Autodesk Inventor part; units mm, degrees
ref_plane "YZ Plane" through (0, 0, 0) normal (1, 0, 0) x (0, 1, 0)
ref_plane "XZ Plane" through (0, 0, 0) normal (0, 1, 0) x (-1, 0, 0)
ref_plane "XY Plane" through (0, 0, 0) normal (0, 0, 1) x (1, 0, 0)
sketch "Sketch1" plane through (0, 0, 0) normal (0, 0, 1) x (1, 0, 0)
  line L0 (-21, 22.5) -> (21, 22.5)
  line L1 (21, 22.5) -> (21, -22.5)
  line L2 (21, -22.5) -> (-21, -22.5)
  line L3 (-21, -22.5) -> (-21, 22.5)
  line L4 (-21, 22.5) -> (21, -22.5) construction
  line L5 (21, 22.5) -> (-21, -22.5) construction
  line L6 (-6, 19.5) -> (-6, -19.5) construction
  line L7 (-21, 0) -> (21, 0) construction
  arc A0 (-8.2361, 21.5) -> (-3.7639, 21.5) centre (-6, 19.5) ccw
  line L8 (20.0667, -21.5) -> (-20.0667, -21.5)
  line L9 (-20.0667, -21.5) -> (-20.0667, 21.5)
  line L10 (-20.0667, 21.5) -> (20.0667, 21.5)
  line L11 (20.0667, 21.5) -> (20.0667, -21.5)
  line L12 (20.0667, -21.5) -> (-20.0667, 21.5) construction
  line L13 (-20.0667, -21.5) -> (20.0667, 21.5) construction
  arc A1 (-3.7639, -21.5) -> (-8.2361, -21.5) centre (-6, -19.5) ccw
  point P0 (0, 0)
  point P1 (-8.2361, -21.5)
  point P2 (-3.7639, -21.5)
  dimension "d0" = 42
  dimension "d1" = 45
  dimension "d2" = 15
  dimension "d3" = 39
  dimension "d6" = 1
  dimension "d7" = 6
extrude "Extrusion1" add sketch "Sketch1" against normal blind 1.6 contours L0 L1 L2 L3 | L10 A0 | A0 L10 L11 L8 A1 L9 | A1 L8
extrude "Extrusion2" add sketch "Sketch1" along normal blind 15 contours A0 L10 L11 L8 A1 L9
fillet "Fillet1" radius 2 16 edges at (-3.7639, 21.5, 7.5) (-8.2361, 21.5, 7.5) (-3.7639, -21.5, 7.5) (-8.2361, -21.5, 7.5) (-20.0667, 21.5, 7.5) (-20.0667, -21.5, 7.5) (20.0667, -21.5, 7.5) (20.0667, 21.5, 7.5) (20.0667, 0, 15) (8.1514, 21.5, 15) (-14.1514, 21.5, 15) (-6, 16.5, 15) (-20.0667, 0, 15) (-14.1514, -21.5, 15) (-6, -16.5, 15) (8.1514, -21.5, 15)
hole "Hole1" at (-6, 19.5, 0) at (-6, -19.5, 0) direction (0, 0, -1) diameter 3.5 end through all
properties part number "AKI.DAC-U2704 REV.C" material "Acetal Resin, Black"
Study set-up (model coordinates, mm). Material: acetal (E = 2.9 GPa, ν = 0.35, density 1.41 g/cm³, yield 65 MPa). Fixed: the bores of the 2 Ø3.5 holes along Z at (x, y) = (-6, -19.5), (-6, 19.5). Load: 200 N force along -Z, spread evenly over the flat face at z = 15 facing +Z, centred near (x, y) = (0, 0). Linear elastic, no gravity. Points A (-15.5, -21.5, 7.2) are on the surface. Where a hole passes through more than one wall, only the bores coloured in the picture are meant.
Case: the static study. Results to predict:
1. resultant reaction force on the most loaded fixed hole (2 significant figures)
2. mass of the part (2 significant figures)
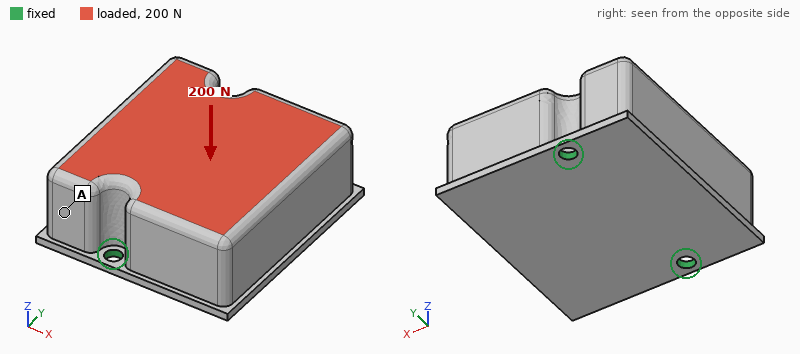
110 N
39 g
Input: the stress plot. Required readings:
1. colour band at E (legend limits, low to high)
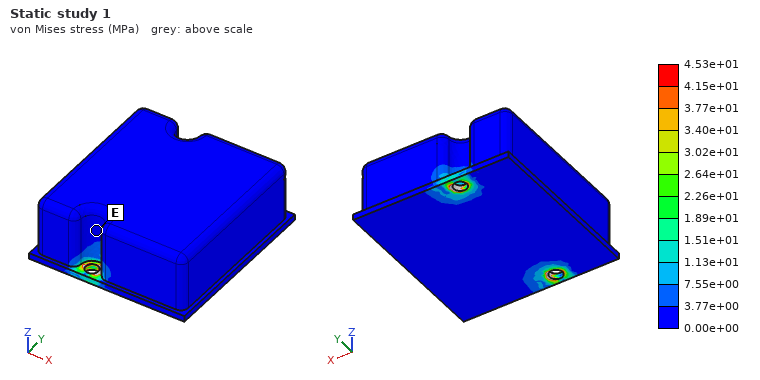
0.00e+00 to 3.77e+00 MPa
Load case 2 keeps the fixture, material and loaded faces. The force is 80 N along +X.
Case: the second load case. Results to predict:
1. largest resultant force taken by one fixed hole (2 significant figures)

40 N
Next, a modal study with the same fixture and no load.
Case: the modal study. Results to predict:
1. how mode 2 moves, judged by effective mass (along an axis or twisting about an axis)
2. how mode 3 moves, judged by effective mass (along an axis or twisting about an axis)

along Z
along Y
